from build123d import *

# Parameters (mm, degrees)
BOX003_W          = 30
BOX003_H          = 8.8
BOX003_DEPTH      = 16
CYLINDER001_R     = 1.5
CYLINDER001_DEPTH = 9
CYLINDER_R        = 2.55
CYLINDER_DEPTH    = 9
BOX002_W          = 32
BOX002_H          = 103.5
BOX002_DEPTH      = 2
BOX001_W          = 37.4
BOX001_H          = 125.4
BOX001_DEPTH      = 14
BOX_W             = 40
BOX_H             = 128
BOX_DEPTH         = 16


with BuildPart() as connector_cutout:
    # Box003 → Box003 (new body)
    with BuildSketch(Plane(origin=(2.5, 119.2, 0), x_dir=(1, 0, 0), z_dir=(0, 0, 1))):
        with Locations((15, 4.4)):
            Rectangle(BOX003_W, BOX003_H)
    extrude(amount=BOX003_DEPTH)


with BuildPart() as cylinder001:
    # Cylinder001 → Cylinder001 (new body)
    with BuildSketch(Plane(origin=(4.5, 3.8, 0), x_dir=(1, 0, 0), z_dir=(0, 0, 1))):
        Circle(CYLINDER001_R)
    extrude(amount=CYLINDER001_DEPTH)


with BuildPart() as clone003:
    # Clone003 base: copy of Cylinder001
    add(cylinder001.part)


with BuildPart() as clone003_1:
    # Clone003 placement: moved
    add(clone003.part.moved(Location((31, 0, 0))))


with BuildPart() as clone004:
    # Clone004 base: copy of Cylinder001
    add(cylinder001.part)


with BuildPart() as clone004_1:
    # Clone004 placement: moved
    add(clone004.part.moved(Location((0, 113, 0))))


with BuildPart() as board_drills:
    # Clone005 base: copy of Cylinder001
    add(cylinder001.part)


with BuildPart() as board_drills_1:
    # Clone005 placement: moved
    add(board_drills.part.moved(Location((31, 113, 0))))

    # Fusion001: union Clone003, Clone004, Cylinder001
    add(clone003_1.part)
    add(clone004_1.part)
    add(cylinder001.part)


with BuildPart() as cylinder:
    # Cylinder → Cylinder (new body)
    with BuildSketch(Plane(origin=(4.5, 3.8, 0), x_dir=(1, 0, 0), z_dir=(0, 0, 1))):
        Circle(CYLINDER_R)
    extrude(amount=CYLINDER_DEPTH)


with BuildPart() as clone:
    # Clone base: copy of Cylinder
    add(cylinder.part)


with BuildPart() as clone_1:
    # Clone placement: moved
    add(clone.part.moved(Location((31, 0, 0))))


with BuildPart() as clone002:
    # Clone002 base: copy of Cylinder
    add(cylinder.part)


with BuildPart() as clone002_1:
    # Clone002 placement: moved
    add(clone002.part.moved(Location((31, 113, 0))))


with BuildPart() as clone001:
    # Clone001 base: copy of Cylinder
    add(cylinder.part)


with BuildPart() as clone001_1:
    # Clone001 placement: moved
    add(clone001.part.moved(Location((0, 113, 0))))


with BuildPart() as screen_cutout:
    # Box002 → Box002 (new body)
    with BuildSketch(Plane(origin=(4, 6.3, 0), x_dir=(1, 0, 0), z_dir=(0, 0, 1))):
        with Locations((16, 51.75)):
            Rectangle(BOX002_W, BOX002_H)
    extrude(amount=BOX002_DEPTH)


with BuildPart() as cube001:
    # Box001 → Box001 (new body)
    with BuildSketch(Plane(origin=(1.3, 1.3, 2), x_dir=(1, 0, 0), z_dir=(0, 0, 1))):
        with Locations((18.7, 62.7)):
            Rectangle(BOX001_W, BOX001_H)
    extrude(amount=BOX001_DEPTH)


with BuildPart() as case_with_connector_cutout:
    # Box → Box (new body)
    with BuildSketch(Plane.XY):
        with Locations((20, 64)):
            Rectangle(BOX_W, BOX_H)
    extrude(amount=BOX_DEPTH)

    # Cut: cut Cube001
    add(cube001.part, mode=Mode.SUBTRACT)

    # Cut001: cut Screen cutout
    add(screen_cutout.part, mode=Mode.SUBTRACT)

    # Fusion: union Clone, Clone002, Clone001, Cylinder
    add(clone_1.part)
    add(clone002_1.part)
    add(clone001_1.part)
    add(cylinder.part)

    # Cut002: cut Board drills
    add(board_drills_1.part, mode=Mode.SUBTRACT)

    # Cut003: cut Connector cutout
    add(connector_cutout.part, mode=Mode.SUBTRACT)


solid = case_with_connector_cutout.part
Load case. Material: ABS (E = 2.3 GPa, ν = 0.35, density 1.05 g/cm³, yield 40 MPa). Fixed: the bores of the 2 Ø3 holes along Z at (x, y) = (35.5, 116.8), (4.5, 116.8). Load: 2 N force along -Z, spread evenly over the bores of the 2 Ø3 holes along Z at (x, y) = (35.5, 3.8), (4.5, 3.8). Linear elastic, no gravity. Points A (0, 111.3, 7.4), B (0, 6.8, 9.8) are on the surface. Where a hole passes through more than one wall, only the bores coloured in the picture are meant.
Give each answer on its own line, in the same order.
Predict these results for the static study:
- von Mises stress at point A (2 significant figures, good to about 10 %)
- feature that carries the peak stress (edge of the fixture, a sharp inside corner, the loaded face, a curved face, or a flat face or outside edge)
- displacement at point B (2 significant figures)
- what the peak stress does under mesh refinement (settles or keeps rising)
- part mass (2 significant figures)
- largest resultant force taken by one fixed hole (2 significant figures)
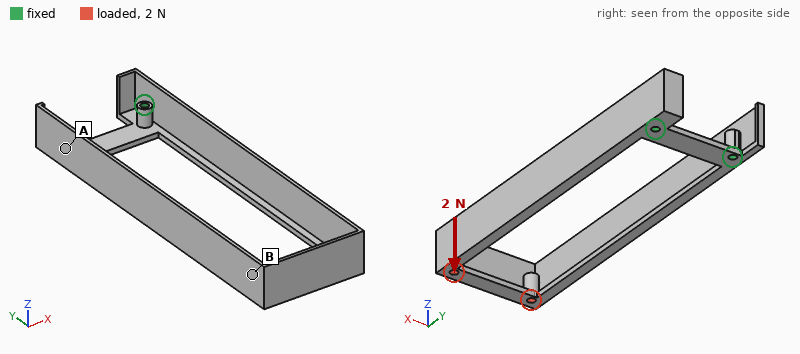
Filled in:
1.0 MPa
a sharp inside corner
1.5 mm
keeps rising
9.3 g
1.2 N
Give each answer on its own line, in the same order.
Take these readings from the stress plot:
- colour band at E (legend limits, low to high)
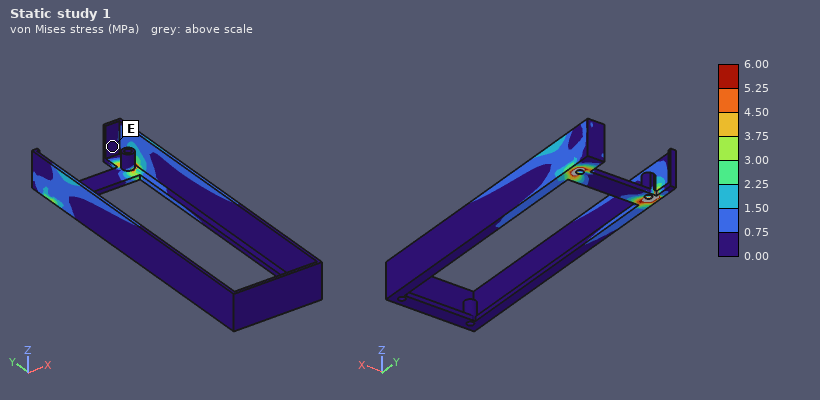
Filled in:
0.00 to 0.75 MPa
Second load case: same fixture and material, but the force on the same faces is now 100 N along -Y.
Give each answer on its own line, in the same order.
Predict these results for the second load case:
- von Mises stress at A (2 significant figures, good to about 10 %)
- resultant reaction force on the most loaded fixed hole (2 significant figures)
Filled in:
3.0 MPa
51 N
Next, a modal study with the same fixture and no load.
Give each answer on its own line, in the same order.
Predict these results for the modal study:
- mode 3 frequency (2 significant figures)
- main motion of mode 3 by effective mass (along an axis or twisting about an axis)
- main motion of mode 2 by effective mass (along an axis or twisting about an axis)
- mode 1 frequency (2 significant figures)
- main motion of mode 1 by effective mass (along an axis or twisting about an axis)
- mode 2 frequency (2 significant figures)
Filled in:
150 Hz
twisting about Y
along Z
67 Hz
along X
100 Hz
